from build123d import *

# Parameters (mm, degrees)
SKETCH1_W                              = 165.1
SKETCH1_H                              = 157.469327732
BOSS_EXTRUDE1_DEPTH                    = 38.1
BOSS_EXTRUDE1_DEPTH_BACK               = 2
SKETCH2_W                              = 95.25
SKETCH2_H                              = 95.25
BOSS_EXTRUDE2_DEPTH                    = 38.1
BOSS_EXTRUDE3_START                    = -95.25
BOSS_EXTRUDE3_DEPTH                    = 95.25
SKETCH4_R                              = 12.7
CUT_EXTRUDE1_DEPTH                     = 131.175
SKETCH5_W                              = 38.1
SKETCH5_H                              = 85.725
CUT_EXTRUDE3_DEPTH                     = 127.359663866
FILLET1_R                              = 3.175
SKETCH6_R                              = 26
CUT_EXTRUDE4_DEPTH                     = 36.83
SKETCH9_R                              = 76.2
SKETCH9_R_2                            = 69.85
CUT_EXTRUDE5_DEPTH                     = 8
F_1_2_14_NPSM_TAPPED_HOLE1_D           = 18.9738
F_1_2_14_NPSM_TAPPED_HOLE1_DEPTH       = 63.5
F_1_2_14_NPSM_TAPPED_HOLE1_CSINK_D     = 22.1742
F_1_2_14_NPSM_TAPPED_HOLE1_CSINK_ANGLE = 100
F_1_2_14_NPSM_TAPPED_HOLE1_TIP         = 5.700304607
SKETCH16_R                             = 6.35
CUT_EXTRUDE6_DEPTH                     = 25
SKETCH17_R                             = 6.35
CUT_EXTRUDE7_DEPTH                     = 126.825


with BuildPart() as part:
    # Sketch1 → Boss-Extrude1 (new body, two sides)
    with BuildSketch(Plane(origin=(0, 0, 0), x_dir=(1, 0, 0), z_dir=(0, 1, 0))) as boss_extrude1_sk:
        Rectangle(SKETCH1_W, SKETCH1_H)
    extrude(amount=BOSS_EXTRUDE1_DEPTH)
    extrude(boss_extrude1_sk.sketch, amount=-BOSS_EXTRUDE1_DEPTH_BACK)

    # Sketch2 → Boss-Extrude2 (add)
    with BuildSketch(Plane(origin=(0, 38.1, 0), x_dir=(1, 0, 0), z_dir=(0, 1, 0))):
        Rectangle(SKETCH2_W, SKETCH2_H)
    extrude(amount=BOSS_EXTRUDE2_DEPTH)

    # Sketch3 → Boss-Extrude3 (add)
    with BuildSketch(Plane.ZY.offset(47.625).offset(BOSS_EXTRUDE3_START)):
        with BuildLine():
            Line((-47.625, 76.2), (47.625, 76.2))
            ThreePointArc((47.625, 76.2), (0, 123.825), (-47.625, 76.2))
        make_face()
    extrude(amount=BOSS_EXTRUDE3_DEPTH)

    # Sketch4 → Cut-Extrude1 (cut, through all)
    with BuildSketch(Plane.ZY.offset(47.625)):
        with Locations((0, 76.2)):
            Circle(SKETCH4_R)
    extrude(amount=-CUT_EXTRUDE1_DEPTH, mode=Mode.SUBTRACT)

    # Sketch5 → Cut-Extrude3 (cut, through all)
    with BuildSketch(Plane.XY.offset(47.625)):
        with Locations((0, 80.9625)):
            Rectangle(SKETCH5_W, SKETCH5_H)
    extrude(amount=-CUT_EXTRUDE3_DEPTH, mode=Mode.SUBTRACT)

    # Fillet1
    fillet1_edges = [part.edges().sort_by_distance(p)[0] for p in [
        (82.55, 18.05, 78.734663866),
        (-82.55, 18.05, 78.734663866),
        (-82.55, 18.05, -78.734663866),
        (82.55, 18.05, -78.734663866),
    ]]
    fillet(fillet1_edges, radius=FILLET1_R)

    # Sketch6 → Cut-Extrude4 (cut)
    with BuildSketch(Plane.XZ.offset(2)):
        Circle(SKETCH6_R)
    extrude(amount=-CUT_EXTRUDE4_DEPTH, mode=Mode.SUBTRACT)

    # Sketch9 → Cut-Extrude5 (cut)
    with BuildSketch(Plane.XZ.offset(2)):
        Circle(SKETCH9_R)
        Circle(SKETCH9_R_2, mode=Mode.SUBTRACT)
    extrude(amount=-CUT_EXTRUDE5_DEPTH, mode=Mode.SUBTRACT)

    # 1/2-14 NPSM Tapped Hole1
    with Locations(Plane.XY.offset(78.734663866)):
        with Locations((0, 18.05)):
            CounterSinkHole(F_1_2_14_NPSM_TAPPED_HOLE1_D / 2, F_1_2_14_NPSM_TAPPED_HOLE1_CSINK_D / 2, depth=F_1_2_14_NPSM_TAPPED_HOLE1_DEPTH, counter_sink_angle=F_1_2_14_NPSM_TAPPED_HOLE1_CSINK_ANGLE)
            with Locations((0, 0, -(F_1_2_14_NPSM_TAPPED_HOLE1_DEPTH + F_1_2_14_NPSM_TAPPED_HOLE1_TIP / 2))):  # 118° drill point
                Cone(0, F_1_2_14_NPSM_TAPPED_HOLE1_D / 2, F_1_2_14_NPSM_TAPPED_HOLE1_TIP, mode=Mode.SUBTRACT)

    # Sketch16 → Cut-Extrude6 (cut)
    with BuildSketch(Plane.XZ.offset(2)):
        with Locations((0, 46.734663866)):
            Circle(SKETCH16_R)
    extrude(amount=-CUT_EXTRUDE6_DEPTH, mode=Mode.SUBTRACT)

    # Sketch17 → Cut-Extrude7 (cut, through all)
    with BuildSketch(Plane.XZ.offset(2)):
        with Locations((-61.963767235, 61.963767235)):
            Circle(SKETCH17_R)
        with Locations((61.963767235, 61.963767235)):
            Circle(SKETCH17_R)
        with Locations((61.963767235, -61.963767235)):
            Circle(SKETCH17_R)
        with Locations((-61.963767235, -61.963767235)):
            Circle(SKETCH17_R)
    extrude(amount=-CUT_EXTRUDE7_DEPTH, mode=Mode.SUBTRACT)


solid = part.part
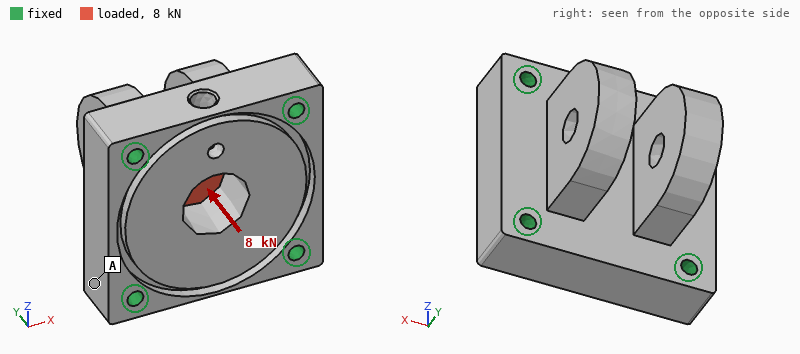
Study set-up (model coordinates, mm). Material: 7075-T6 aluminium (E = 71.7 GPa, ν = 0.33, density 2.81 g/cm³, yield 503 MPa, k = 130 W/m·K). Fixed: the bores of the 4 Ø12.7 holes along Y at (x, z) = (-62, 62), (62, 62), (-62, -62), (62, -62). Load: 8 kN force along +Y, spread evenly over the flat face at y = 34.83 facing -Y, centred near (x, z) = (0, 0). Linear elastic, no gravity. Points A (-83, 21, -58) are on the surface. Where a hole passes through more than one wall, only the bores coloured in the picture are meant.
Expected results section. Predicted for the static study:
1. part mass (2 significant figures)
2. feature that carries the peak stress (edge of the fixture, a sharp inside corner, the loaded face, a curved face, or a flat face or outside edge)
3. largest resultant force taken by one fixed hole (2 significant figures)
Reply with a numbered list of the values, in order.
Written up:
1. 3.6 kg
2. a flat face or outside edge
3. 2.0 kN
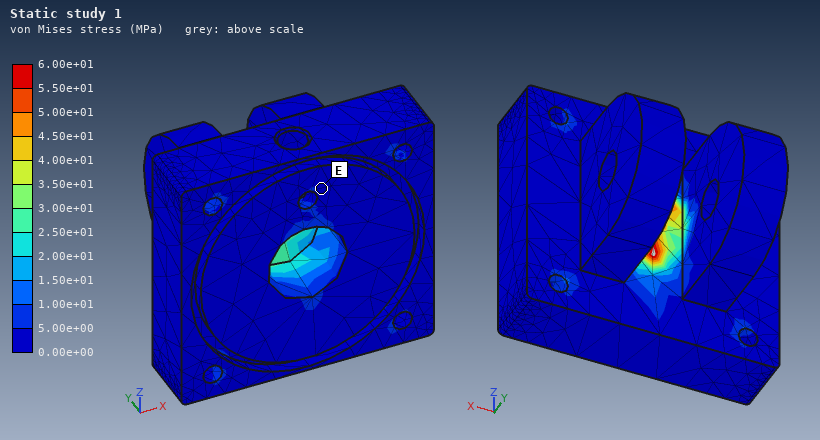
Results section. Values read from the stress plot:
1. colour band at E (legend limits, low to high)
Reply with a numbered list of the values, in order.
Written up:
1. 0.00e+00 to 5.00e+00 MPa
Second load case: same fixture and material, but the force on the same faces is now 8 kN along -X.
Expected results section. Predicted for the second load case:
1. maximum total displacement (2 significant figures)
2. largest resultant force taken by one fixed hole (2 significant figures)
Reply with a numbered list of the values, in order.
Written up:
1. 6.2 µm
2. 2.3 kN
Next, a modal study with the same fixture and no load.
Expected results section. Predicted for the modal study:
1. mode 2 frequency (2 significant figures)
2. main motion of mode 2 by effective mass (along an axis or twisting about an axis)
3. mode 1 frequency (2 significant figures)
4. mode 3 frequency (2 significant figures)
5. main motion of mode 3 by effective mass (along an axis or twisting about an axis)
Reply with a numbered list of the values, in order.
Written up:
1. 2700 Hz
2. along X
3. 2500 Hz
4. 4700 Hz
5. along Z
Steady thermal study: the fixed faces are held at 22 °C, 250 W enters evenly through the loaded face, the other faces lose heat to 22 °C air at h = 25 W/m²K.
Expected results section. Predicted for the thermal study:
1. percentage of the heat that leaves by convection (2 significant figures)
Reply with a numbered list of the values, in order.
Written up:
1. 9.4 %
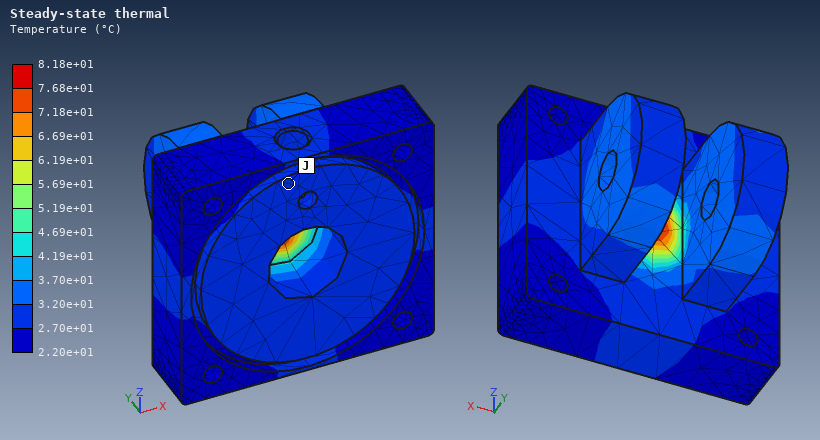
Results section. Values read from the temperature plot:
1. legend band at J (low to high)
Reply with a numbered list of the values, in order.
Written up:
1. 2.70e+01 to 3.20e+01 °C
